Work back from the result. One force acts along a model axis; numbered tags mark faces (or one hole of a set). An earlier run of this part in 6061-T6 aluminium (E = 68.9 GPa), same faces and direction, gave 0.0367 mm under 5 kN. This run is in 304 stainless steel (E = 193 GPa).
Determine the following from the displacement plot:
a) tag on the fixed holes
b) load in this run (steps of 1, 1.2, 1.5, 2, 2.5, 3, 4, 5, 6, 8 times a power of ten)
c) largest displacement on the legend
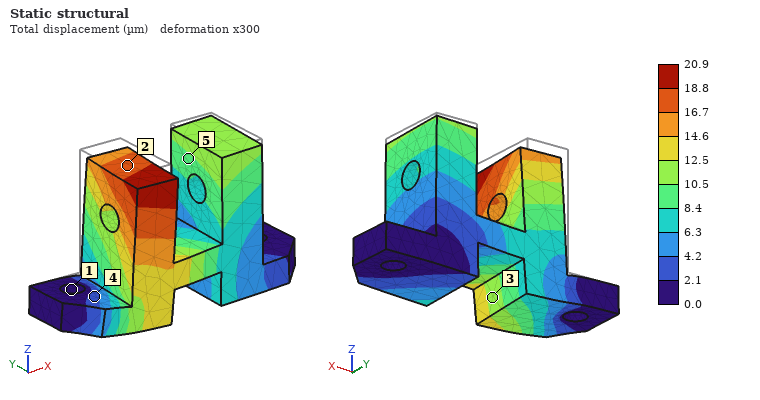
1
8 kN
20.9 µm
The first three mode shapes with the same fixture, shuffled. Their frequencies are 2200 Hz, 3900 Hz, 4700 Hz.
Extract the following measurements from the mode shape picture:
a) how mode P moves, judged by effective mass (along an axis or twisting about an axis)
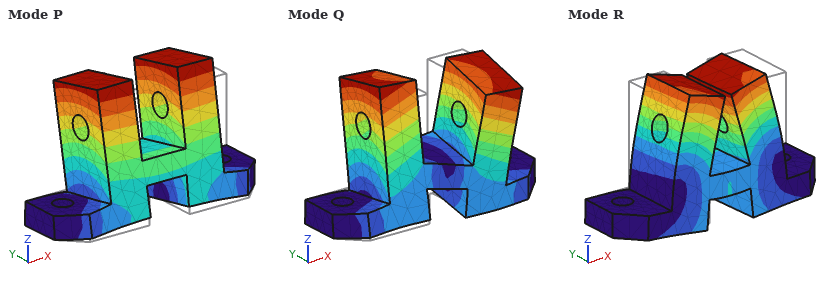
along Y
